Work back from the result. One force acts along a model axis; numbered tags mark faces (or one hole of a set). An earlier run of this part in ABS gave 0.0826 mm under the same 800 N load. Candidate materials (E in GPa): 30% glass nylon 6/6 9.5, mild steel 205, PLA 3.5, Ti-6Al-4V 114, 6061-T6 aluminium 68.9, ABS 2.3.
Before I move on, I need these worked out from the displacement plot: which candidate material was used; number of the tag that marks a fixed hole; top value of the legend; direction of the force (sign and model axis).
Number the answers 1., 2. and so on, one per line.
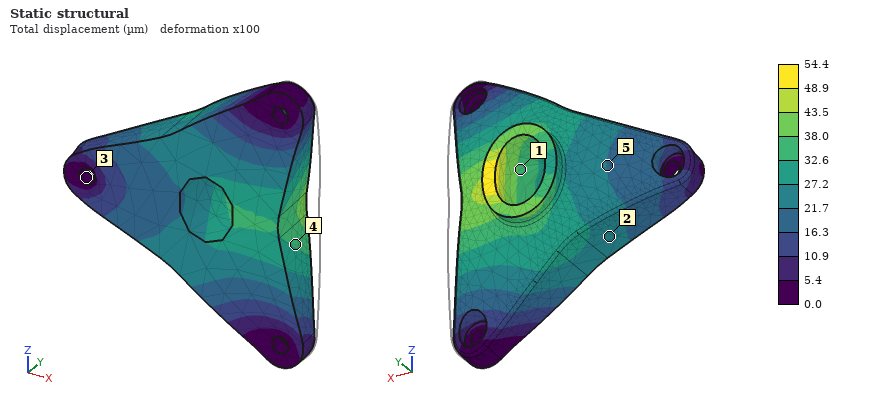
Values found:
1. PLA
2. 3
3. 54.4 µm
4. -X
